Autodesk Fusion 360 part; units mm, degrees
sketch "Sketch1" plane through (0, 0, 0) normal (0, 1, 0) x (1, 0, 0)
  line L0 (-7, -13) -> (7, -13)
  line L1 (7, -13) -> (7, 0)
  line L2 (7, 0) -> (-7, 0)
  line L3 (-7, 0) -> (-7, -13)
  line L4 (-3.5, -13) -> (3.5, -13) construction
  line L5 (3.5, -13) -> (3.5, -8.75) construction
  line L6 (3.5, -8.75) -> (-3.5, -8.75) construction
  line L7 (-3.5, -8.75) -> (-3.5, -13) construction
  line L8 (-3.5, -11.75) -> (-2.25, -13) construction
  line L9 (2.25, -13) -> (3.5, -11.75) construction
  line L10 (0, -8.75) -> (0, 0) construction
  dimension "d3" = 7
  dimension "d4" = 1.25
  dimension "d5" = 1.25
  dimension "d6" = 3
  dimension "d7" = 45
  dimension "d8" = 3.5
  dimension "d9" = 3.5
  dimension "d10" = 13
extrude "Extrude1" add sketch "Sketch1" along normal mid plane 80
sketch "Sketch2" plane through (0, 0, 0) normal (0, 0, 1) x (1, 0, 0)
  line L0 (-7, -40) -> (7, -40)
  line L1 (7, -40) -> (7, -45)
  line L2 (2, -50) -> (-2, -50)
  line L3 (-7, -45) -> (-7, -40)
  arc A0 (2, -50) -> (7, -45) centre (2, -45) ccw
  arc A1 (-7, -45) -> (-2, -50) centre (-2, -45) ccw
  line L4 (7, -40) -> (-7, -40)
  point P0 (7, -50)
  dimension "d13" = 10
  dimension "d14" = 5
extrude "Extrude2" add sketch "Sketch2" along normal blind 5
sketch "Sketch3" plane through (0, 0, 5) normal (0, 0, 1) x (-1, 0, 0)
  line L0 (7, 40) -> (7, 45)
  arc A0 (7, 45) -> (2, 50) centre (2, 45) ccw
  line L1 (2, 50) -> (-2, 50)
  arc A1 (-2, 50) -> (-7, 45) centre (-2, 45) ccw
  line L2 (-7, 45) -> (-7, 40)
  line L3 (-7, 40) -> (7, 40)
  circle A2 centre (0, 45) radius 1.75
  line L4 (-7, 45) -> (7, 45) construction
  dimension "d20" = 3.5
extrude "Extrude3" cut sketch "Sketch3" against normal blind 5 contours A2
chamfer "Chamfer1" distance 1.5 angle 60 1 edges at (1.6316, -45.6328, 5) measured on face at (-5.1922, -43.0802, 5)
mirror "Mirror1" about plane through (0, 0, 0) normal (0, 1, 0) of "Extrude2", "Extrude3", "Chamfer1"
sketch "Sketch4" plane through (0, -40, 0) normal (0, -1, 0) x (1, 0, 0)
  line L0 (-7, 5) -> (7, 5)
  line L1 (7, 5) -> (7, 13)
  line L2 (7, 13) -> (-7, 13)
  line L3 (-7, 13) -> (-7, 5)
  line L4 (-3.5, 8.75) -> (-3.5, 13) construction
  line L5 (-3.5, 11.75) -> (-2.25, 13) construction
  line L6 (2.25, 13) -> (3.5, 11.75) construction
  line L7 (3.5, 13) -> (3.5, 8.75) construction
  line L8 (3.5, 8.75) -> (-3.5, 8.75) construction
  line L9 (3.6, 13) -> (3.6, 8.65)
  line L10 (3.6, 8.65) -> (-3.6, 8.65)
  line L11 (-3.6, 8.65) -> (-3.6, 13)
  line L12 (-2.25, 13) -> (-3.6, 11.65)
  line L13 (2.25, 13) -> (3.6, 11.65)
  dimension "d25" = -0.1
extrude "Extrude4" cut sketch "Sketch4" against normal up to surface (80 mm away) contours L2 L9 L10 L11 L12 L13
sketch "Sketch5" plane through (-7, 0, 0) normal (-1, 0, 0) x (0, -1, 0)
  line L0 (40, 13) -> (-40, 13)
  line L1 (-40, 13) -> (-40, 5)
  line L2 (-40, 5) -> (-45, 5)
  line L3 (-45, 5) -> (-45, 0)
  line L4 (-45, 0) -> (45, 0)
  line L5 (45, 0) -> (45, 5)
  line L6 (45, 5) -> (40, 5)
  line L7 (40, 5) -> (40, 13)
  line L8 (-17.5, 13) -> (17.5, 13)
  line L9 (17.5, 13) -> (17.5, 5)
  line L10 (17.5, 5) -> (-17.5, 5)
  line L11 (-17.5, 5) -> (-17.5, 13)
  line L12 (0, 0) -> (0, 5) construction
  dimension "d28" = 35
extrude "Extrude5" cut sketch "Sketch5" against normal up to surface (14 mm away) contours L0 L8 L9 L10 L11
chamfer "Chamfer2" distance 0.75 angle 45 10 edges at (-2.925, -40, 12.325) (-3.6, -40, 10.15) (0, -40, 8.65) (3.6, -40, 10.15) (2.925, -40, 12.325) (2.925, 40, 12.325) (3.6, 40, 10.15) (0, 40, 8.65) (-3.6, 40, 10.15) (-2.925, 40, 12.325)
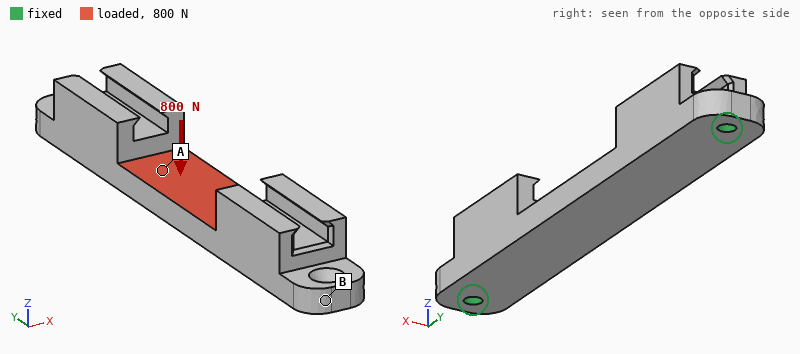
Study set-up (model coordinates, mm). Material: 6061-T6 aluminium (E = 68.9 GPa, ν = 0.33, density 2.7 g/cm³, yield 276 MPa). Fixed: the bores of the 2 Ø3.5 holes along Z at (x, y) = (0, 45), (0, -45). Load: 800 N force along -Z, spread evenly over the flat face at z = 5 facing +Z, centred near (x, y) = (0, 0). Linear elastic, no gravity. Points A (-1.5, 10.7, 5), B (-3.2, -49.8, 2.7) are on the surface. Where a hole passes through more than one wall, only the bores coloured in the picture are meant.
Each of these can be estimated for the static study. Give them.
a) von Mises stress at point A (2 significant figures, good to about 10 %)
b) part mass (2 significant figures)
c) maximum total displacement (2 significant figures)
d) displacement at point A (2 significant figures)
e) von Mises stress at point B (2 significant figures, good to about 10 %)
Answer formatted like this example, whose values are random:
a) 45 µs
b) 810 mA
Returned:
a) 91 MPa
b) 28 g
c) 0.33 mm
d) 0.29 mm
e) 45 MPa
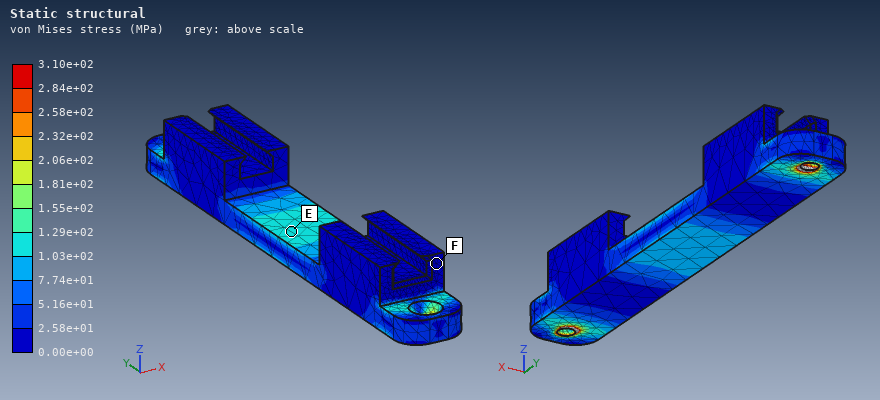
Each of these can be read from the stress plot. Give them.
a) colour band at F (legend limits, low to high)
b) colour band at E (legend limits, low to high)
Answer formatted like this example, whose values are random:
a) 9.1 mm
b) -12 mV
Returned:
a) 0.00e+00 to 2.58e+01 MPa
b) 1.03e+02 to 1.29e+02 MPa
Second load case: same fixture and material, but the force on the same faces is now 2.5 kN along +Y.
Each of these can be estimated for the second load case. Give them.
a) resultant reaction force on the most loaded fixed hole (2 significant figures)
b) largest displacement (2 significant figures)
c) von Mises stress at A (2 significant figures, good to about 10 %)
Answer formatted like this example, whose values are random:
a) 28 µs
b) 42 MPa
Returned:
a) 1.3 kN
b) 13 µm
c) 27 MPa
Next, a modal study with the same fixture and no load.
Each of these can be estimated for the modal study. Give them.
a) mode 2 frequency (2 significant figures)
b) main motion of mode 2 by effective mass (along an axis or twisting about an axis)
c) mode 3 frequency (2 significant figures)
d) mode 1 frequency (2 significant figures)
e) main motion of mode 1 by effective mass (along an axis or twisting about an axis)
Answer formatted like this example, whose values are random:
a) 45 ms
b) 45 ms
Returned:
a) 4600 Hz
b) along X
c) 6800 Hz
d) 2400 Hz
e) along Z
